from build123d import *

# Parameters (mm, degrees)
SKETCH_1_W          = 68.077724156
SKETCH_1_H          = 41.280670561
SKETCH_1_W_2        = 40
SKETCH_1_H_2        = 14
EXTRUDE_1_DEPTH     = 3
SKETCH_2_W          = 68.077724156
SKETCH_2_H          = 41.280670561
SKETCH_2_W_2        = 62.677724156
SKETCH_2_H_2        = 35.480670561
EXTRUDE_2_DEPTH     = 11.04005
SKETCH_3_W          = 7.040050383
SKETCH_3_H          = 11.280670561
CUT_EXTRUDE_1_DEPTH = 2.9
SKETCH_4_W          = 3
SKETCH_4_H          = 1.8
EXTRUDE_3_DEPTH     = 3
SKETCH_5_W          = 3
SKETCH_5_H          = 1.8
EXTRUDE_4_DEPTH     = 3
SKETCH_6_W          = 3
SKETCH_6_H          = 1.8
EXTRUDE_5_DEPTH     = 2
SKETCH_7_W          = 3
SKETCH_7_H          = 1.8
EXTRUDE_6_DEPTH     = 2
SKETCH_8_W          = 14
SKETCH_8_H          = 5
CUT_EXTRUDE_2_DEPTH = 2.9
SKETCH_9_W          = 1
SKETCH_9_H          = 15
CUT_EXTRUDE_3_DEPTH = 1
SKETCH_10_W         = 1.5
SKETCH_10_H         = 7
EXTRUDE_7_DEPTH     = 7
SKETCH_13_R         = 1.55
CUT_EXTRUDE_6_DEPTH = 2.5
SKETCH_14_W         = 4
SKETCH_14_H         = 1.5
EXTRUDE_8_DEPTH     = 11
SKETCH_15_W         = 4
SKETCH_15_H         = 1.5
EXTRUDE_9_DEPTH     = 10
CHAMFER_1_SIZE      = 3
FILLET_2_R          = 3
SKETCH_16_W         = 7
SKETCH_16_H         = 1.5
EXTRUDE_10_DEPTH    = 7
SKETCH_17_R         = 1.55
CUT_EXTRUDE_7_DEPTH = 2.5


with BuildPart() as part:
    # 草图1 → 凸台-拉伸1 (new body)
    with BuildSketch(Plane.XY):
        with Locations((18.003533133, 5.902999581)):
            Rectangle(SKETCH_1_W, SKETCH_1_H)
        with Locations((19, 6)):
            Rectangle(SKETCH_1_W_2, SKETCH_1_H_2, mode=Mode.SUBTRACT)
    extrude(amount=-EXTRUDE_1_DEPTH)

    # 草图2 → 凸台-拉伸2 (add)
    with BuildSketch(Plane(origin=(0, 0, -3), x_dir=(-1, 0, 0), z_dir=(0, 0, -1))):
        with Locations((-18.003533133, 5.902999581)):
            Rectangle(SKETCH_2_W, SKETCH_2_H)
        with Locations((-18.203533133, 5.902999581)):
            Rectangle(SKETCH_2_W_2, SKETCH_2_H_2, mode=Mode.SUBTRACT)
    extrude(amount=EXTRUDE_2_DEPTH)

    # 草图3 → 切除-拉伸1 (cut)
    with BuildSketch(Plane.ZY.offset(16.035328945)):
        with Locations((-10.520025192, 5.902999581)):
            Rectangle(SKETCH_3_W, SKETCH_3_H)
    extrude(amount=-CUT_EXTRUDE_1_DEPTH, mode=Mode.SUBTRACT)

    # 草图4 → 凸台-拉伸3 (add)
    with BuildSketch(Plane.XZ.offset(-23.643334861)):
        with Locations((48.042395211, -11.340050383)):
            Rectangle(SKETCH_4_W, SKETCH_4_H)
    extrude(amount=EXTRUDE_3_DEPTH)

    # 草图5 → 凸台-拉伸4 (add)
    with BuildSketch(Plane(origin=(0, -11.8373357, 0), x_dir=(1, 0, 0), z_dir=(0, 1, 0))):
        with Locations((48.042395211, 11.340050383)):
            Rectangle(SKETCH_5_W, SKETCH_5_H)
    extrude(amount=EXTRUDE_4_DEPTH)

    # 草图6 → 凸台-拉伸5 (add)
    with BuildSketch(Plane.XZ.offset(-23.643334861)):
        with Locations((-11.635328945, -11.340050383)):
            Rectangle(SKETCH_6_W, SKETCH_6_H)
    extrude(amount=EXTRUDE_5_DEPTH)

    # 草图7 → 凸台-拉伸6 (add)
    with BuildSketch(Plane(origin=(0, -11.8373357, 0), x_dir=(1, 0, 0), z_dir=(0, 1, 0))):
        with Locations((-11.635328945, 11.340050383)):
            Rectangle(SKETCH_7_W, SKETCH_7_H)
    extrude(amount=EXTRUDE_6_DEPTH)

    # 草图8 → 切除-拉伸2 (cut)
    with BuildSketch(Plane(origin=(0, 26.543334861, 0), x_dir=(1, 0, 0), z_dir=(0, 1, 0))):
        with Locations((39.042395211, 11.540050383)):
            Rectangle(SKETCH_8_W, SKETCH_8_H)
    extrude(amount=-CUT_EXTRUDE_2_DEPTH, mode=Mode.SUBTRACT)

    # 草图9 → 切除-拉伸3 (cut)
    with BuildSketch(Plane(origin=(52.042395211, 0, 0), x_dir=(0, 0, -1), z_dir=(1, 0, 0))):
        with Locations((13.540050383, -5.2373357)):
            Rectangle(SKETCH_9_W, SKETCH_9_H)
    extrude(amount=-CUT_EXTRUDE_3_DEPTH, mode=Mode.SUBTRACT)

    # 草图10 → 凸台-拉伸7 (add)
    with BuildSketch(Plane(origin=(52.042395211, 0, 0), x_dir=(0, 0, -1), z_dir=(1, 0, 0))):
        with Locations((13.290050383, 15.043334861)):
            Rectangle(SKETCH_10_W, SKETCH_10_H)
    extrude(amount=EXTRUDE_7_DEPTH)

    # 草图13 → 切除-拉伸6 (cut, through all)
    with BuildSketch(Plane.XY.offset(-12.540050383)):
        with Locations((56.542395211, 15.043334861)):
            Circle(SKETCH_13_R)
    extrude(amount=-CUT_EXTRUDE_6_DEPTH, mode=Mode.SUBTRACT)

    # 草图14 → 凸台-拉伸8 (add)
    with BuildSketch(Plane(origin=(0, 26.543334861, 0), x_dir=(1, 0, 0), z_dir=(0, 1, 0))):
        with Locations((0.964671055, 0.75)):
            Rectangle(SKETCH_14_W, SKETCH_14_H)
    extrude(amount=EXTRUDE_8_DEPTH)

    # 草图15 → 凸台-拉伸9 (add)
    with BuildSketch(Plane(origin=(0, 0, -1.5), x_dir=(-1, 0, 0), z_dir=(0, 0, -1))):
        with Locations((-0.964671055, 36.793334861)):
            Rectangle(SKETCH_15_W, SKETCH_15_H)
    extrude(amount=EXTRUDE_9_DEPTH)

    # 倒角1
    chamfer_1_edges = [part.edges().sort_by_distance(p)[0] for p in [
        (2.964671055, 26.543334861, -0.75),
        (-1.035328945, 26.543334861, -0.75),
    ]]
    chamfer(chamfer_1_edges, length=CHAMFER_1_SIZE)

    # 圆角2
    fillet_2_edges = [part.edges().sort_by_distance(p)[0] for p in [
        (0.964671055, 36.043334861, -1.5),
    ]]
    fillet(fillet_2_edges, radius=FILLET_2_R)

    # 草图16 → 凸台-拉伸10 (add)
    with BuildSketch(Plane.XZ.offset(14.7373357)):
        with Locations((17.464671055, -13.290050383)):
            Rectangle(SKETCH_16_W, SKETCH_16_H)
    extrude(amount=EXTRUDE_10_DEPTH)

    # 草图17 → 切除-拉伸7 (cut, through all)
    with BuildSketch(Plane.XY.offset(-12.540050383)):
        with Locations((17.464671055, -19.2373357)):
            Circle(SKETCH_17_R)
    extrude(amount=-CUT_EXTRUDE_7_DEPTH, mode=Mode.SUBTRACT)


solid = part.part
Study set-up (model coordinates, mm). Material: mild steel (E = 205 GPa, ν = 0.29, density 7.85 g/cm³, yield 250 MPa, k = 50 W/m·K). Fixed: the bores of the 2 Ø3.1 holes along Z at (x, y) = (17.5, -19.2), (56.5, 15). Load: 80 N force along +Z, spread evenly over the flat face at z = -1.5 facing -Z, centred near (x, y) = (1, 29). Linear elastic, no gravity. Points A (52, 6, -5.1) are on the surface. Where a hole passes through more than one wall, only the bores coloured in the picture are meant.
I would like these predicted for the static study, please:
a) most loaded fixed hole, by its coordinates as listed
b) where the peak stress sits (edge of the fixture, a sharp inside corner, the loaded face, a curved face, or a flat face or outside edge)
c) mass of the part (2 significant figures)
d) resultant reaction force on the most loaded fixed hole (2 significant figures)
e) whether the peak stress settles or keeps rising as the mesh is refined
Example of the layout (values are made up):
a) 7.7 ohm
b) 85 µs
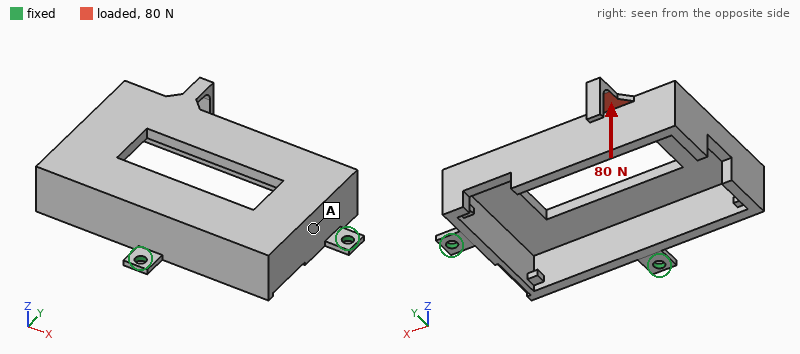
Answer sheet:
a) (17.5, -19.2)
b) edge of the fixture
c) 100 g
d) 73 N
e) keeps rising
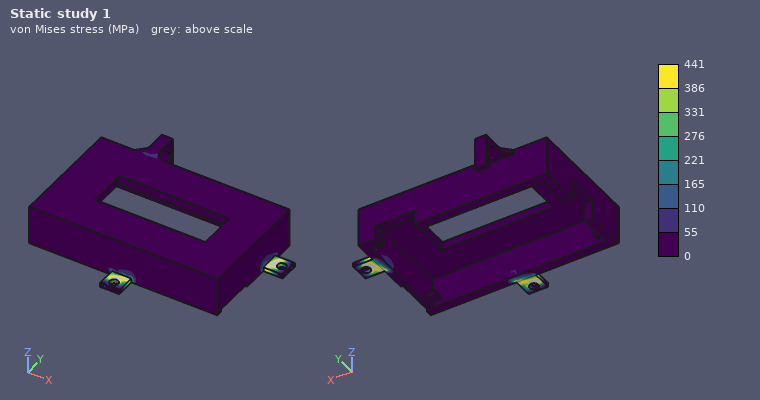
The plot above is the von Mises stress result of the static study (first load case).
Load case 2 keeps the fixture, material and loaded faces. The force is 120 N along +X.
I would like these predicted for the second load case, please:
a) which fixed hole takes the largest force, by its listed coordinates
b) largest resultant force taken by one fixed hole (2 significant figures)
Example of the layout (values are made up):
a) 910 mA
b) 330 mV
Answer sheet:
a) (56.5, 15)
b) 120 N
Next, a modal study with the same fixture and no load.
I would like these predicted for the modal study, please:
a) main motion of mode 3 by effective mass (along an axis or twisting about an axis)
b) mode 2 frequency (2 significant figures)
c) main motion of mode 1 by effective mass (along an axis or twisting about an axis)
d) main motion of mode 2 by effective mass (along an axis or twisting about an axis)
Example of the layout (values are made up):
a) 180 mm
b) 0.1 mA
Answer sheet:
a) along X
b) 1600 Hz
c) along Z
d) along Y
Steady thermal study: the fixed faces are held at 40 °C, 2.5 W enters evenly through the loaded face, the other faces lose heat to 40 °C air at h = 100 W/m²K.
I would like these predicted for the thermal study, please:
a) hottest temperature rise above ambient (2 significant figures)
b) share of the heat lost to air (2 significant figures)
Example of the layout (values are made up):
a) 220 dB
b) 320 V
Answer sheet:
a) 23 K
b) 96 %
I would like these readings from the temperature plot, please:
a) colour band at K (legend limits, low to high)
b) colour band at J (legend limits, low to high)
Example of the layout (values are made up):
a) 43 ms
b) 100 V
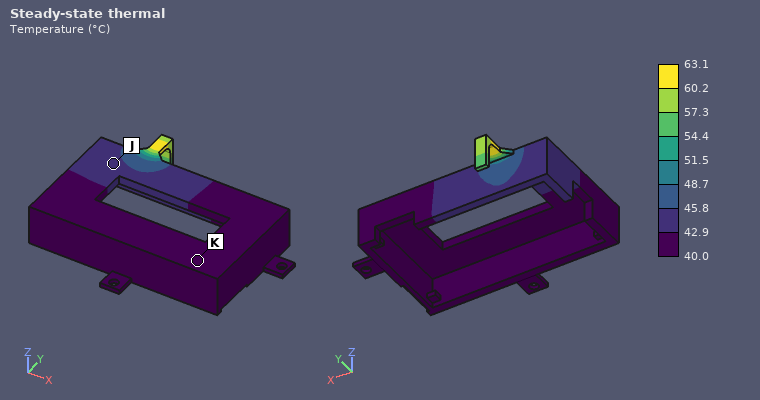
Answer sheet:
a) 40.0 to 42.9 °C
b) 42.9 to 45.8 °C
